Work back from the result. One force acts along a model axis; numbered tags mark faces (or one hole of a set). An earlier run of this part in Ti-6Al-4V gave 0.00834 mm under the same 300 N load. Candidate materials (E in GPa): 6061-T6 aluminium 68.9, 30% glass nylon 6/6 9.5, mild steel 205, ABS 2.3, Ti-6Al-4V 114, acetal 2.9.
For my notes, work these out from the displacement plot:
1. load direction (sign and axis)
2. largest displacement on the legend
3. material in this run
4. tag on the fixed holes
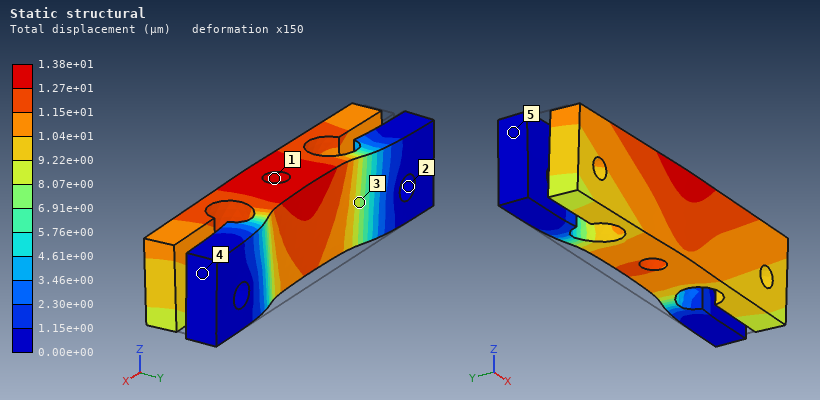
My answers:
-Y
1.38e+01 µm
6061-T6 aluminium
2
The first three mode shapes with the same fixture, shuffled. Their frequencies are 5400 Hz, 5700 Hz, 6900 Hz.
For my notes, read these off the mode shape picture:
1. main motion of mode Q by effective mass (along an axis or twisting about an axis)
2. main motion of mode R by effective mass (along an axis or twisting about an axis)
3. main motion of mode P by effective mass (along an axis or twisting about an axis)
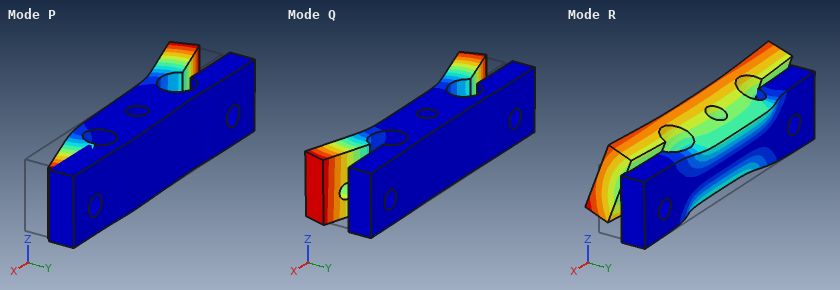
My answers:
along Y
along Z
twisting about Z
